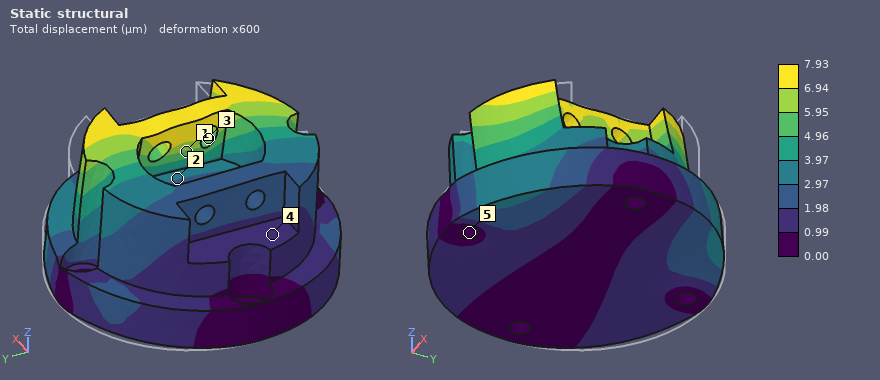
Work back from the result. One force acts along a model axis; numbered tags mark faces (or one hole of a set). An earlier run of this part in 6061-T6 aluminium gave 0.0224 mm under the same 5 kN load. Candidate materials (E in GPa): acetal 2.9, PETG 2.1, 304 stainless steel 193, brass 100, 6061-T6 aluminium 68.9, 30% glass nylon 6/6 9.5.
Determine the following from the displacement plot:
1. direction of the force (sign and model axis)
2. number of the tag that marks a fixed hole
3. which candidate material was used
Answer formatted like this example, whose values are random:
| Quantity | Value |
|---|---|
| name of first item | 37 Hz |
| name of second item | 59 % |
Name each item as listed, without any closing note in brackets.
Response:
| Quantity | Value |
|---|---|
| direction of the force | -Y |
| number of the tag that marks a fixed hole | 5 |
| which candidate material was used | 304 stainless steel |
